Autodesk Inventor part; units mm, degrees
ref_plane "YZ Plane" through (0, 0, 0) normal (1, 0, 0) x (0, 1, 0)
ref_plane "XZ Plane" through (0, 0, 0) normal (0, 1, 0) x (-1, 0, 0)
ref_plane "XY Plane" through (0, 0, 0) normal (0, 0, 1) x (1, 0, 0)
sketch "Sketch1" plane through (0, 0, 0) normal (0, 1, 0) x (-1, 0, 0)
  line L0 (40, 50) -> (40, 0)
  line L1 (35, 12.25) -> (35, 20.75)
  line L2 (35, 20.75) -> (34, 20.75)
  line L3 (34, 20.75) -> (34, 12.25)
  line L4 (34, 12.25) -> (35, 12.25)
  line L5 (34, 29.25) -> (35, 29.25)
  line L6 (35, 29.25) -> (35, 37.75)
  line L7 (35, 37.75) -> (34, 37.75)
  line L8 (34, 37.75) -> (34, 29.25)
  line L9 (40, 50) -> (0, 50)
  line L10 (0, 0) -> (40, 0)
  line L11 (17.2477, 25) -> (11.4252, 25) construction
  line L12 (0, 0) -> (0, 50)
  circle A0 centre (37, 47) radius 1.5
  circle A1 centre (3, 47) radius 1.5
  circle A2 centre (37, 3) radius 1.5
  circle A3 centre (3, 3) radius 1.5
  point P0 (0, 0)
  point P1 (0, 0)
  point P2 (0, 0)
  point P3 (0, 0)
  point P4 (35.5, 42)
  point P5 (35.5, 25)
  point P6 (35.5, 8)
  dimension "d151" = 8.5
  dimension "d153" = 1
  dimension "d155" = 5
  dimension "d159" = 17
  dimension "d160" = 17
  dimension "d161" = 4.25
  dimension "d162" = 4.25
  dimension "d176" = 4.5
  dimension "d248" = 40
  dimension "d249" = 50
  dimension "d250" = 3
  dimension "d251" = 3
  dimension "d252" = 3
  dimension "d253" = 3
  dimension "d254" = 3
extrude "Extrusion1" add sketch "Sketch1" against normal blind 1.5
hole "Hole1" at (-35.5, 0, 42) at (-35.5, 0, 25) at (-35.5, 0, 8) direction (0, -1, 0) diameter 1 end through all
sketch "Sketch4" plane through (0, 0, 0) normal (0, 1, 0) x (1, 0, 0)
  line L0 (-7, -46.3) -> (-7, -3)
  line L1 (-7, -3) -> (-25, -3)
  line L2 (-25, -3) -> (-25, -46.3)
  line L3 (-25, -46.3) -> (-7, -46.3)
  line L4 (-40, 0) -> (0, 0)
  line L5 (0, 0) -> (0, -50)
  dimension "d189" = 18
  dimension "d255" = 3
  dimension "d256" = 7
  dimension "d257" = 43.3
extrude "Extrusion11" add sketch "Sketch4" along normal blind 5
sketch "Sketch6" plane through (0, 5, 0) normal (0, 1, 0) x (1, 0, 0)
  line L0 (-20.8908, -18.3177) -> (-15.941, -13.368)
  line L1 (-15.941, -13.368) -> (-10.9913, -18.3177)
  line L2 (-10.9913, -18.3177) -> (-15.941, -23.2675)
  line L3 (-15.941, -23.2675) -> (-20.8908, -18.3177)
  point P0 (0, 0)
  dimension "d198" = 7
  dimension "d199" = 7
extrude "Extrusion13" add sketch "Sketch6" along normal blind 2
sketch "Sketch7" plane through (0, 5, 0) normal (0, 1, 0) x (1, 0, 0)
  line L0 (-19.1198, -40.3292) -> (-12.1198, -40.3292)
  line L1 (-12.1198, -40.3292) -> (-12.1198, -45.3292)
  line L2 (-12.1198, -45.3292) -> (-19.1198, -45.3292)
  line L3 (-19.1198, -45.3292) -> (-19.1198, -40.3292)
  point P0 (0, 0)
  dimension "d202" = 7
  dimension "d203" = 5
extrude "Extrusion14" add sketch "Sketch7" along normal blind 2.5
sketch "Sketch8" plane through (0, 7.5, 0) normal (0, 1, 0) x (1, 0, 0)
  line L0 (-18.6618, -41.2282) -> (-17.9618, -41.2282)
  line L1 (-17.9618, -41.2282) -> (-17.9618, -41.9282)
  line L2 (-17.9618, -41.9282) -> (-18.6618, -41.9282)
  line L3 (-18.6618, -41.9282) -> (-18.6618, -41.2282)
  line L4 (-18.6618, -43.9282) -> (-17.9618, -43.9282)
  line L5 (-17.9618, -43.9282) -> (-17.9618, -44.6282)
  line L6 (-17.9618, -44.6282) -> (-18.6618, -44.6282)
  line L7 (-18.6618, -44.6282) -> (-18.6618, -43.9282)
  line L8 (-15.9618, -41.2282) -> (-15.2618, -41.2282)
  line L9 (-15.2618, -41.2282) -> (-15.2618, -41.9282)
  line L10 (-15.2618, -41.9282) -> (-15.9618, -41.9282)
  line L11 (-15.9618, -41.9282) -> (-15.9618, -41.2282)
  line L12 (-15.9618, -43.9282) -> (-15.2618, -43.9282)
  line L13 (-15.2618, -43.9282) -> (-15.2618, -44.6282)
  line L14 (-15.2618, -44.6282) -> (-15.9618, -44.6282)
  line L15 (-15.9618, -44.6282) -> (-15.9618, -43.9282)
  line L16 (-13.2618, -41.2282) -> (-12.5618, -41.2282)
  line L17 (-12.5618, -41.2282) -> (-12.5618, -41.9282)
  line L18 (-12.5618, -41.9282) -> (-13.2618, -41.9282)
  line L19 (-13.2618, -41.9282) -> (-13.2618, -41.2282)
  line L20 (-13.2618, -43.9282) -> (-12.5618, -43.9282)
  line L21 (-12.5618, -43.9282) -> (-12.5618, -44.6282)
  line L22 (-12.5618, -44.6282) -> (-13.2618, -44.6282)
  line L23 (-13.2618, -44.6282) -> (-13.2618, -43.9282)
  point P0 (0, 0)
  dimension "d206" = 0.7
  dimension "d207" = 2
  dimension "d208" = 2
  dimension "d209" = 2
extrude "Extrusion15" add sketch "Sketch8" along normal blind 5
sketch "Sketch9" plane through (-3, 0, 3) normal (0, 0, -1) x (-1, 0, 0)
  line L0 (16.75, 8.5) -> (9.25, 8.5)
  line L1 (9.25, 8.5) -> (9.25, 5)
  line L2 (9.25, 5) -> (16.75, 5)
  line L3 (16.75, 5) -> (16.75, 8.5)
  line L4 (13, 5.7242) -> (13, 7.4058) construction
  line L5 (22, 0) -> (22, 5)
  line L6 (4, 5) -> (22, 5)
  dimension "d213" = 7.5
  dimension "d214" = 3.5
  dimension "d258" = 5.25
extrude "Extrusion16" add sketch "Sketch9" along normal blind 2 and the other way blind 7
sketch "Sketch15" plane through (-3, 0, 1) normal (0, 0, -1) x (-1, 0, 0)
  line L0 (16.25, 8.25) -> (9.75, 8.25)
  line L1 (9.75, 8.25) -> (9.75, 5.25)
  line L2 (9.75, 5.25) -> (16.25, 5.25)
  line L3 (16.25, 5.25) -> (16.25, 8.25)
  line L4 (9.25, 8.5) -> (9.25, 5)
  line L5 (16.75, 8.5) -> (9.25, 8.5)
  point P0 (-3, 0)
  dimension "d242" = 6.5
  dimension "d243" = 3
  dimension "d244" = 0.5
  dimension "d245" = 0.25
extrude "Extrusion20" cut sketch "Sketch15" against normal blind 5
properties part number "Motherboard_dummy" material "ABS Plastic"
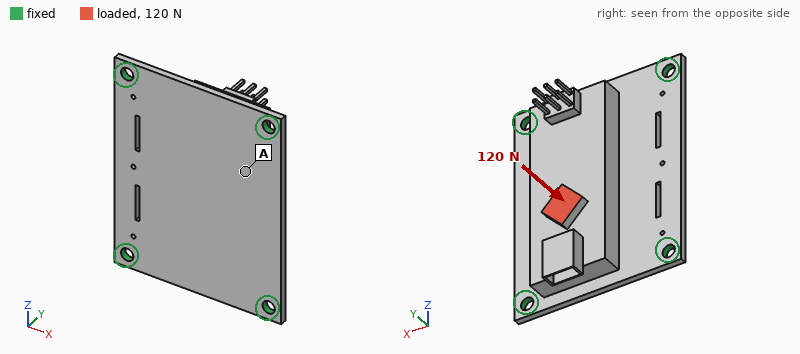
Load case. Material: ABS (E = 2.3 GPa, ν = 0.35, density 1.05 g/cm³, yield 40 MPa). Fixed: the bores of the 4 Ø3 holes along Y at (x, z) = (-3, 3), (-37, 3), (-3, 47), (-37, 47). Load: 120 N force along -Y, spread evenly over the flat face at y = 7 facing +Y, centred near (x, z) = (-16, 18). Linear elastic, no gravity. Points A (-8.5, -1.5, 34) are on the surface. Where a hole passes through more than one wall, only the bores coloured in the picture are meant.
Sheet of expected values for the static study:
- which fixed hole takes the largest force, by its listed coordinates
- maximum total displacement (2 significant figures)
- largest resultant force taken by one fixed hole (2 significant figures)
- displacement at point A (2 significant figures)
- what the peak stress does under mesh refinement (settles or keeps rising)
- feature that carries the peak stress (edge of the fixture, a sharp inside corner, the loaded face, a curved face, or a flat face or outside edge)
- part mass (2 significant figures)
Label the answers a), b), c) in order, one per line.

a) (-3, 3)
b) 0.46 mm
c) 72 N
d) 0.17 mm
e) keeps rising
f) edge of the fixture
g) 7.5 g
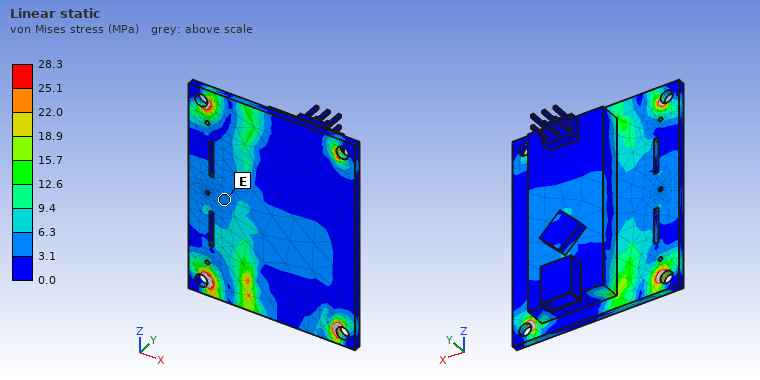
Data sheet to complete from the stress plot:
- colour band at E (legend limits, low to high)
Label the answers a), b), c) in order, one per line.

a) 3.1 to 6.3 MPa
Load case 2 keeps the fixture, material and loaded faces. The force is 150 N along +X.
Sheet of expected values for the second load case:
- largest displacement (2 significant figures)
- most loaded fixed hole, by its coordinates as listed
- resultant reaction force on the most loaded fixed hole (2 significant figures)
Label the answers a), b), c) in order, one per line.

a) 0.36 mm
b) (-3, 3)
c) 61 N
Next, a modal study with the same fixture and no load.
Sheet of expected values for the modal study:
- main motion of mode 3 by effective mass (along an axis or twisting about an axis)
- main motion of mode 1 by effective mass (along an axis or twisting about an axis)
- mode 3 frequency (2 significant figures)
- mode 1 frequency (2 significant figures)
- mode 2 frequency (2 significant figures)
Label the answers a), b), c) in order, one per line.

a) twisting about X
b) along Y
c) 2600 Hz
d) 1200 Hz
e) 2400 Hz
